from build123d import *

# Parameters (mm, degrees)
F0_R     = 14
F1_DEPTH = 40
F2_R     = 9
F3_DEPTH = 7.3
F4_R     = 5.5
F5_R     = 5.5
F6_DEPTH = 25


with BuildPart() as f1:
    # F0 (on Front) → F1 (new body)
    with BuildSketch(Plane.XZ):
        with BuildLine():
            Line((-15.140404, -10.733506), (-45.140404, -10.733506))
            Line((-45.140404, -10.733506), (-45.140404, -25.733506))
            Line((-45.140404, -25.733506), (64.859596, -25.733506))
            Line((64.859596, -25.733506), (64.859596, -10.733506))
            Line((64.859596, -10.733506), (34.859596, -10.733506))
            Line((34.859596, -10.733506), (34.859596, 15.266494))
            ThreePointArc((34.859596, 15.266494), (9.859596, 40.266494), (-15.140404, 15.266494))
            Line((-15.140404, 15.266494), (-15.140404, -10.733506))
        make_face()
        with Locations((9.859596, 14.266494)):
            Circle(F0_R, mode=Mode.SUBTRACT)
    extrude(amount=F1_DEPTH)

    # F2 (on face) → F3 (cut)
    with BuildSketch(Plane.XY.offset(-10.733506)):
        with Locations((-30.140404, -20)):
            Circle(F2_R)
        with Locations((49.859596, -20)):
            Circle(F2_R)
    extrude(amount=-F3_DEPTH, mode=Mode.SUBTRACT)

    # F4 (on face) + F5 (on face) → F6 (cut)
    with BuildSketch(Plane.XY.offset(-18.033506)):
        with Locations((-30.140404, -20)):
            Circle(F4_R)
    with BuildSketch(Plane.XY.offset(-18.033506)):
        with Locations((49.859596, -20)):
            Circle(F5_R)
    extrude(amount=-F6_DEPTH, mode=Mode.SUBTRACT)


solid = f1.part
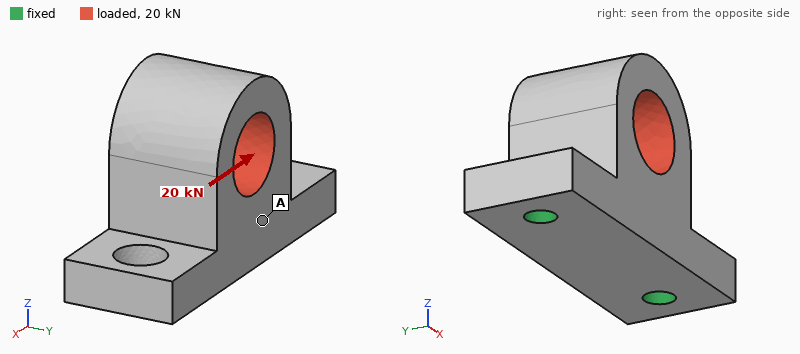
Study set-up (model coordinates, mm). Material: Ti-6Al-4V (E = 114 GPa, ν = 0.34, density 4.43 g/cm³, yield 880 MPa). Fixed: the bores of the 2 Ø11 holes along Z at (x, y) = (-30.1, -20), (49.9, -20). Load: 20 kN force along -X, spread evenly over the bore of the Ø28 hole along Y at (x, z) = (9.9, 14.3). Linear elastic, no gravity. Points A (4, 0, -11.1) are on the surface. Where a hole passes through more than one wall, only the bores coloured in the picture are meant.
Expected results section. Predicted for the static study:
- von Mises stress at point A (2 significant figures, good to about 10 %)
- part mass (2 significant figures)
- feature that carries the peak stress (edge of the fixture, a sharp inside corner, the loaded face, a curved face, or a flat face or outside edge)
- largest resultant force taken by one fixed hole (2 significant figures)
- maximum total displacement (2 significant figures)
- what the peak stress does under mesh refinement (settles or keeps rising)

22 MPa
560 g
edge of the fixture
14 kN
69 µm
keeps rising
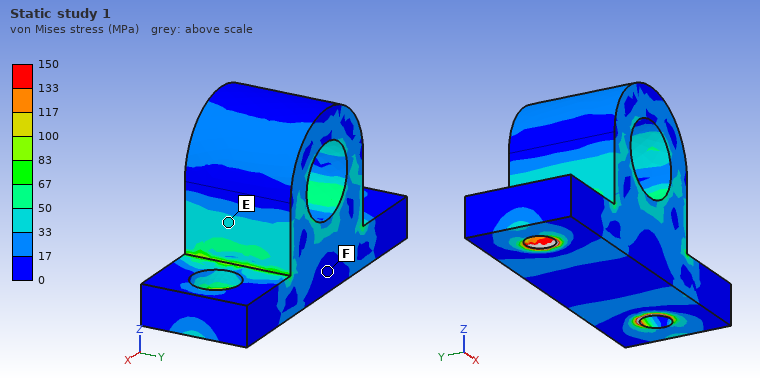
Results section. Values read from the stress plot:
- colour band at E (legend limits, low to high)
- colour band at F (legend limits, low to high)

33 to 50 MPa
0 to 17 MPa
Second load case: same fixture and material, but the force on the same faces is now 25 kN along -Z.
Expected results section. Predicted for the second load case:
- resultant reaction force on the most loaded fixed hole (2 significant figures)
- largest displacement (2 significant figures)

15 kN
36 µm
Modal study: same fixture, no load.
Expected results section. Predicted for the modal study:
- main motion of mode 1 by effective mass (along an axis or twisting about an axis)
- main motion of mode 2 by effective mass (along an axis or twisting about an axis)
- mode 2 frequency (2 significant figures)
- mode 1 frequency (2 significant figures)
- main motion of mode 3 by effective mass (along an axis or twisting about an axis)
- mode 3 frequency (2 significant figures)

along Y
along X
5800 Hz
2200 Hz
along Z
6800 Hz
